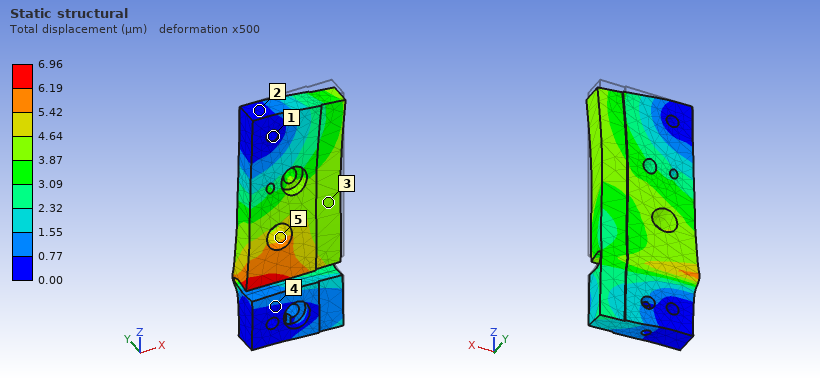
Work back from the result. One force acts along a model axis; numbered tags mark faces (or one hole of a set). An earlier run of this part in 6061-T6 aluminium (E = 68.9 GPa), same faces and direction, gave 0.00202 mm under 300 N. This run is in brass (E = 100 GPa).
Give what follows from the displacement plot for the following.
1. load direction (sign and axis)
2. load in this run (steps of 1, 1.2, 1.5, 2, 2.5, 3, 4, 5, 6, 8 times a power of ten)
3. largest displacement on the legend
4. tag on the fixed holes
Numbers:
-Z
1.5 kN
6.96 µm
1
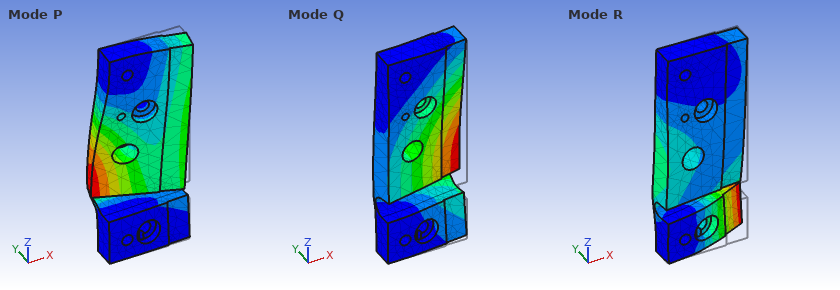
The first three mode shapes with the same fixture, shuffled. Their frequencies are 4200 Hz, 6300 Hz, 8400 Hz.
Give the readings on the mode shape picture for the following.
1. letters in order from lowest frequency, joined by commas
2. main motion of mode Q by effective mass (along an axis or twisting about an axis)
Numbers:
Q, P, R
along Y
